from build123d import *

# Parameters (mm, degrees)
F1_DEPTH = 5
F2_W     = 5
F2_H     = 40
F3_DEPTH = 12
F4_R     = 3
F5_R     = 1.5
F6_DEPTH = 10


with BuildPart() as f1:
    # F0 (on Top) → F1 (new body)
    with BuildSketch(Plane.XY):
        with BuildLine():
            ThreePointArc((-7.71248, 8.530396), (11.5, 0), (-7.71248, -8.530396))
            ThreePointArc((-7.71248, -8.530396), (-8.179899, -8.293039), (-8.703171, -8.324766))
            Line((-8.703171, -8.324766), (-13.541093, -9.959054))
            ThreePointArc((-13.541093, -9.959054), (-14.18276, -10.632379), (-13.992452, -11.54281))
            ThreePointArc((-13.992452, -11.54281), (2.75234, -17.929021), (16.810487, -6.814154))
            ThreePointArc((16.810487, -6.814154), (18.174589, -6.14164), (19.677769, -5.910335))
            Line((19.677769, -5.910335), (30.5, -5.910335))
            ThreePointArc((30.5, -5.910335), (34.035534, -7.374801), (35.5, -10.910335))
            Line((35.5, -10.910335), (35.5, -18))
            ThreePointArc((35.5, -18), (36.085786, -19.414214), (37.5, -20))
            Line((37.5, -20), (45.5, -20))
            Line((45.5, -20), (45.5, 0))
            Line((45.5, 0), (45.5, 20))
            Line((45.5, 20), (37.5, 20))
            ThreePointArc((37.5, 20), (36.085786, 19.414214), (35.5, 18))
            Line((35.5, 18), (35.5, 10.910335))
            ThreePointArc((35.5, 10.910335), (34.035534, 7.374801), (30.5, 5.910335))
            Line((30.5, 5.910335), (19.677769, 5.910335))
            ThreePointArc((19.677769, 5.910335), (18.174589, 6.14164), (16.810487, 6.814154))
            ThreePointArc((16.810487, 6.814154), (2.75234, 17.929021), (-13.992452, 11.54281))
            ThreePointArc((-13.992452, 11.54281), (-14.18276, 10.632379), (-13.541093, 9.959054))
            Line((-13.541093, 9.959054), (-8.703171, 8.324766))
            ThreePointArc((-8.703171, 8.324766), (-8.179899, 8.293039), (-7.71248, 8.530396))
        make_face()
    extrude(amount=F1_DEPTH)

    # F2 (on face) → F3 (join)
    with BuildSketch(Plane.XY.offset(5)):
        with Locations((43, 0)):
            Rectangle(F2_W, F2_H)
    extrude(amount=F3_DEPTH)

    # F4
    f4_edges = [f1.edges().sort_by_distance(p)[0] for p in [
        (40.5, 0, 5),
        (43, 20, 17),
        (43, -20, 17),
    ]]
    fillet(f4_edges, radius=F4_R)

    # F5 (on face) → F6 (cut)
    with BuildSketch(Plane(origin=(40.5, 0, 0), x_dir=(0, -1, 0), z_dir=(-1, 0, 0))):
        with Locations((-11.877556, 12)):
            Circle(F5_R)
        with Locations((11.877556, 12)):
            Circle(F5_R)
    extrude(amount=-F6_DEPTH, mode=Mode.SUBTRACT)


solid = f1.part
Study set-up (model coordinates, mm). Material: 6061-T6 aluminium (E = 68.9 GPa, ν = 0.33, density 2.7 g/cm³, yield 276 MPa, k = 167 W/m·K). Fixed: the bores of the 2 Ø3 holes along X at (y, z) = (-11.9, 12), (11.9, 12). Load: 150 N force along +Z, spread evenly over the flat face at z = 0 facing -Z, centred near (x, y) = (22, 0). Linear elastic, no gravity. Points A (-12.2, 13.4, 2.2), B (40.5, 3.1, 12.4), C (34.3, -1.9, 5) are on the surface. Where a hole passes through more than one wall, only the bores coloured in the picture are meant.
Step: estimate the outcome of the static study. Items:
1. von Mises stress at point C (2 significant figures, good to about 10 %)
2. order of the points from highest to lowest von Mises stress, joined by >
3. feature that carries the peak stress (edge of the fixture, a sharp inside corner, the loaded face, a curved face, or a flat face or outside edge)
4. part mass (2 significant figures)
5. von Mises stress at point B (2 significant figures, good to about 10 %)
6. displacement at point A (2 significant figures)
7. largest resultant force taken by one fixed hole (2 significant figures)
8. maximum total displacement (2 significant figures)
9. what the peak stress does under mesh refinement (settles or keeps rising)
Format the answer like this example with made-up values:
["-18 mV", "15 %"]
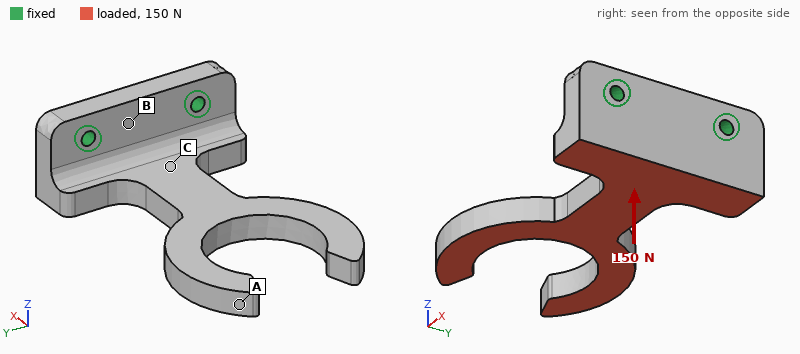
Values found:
["37 MPa", "C > B > A", "edge of the fixture", "21 g", "7.6 MPa", "0.27 mm", "85 N", "0.28 mm", "keeps rising"]
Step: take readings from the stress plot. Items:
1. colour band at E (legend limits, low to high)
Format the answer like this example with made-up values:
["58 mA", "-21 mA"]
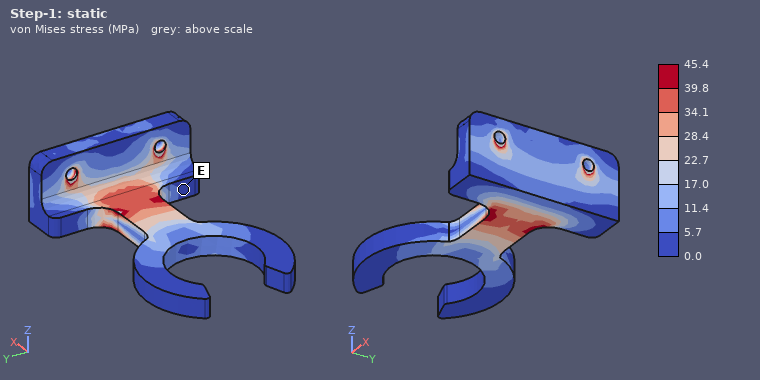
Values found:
["0.0 to 5.7 MPa"]
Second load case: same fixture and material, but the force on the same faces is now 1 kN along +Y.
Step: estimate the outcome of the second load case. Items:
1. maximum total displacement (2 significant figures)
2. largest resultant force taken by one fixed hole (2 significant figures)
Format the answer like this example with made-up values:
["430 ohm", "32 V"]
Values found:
["0.38 mm", "1.1 kN"]
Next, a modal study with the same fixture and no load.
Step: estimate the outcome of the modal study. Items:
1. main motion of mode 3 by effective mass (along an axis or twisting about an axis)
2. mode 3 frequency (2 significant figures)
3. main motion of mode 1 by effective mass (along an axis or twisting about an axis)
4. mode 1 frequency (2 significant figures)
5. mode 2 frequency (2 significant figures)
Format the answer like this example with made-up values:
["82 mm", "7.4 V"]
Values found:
["along Y", "2600 Hz", "along Z", "1200 Hz", "2500 Hz"]
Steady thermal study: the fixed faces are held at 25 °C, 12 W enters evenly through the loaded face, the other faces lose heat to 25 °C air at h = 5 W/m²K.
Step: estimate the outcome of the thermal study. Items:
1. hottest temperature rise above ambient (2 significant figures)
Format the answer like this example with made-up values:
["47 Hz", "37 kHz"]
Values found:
["26 K"]
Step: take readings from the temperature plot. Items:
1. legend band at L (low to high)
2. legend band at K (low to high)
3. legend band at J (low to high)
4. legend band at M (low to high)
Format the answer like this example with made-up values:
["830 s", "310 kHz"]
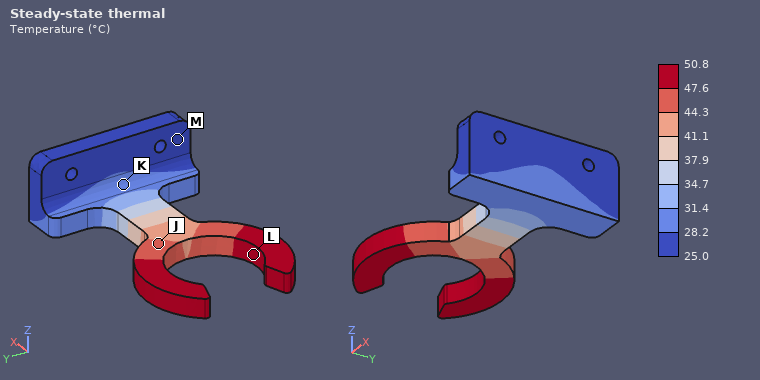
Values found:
["47.6 to 50.8 °C", "28.2 to 31.4 °C", "44.3 to 47.6 °C", "25.0 to 28.2 °C"]
